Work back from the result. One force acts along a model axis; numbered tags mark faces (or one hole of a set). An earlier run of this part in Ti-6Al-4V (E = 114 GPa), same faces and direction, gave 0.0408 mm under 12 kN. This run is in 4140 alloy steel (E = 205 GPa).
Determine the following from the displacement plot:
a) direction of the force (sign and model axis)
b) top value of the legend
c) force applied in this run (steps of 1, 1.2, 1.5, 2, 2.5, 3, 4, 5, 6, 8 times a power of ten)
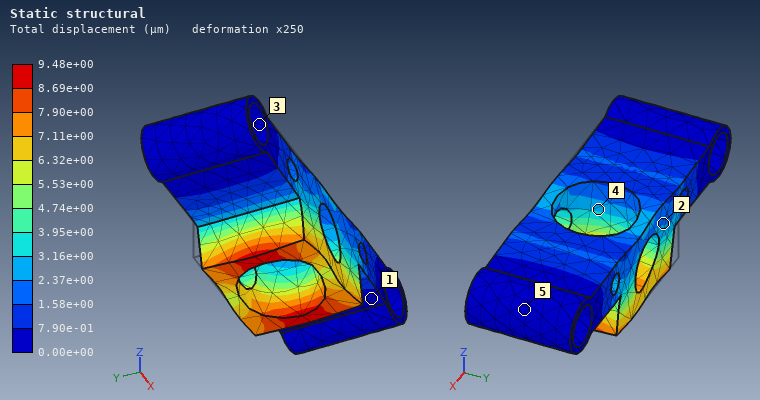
+X
9.48e+00 µm
5 kN
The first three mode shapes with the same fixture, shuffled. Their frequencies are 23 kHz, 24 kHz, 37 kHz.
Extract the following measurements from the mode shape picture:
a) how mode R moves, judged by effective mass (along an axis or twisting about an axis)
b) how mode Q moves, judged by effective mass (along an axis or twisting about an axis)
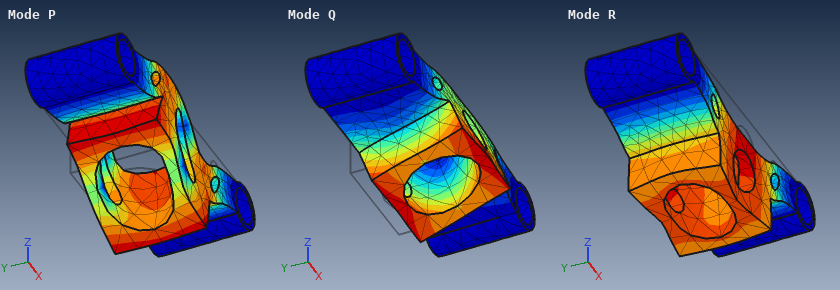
along Z
along Y
